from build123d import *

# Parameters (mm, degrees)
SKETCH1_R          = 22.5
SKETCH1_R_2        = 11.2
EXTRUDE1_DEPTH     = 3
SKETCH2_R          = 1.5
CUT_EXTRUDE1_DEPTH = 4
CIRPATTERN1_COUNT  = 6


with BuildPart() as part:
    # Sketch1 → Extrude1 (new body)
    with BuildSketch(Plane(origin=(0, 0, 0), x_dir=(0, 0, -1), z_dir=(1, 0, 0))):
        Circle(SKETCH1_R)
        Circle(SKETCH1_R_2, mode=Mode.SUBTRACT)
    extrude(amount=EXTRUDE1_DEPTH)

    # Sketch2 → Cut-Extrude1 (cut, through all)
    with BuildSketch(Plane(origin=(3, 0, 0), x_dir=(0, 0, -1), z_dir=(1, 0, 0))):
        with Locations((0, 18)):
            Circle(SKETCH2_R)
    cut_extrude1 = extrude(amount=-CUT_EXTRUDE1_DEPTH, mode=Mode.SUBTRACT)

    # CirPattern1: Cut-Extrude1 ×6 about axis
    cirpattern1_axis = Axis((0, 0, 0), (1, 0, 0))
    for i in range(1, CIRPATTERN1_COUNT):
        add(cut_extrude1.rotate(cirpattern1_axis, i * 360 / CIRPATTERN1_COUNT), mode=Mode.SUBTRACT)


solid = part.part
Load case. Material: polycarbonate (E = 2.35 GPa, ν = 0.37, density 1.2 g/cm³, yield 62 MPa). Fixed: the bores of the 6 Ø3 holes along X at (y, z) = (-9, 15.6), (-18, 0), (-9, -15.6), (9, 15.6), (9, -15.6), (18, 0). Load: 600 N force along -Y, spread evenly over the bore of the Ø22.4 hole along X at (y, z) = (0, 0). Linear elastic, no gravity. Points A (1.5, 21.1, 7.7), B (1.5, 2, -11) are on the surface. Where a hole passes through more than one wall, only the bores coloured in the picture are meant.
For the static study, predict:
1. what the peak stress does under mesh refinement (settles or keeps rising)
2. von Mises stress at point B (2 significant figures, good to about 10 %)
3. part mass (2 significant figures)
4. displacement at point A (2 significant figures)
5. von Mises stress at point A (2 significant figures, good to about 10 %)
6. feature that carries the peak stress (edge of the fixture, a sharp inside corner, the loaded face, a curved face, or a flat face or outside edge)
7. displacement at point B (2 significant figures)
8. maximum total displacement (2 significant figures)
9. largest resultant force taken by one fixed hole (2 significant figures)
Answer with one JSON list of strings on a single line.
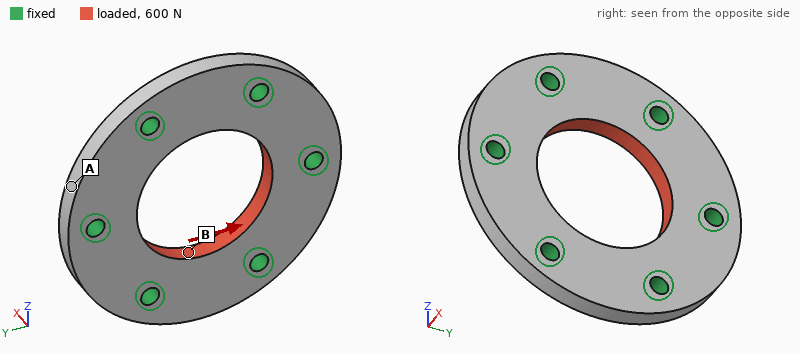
["keeps rising", "4.9 MPa", "4.2 g", "9.6 µm", "1.8 MPa", "edge of the fixture", "14 µm", "18 µm", "130 N"]
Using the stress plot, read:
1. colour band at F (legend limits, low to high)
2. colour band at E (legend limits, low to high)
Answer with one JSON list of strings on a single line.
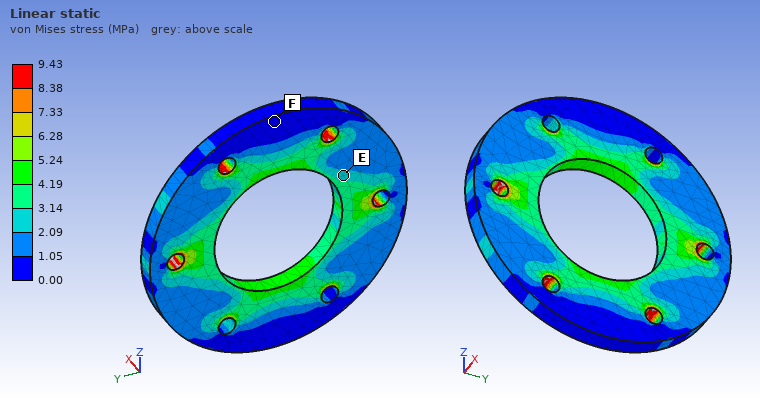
["0.00 to 1.05 MPa", "2.09 to 3.14 MPa"]
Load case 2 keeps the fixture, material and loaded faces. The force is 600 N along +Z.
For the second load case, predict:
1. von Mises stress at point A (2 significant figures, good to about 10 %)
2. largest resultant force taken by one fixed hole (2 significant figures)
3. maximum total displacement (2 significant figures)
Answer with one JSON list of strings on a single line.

["0.95 MPa", "120 N", "19 µm"]
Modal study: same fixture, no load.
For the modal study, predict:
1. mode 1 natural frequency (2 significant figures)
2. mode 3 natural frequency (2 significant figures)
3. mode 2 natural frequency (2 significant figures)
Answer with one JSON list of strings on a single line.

["10000 Hz", "10 kHz", "10 kHz"]
